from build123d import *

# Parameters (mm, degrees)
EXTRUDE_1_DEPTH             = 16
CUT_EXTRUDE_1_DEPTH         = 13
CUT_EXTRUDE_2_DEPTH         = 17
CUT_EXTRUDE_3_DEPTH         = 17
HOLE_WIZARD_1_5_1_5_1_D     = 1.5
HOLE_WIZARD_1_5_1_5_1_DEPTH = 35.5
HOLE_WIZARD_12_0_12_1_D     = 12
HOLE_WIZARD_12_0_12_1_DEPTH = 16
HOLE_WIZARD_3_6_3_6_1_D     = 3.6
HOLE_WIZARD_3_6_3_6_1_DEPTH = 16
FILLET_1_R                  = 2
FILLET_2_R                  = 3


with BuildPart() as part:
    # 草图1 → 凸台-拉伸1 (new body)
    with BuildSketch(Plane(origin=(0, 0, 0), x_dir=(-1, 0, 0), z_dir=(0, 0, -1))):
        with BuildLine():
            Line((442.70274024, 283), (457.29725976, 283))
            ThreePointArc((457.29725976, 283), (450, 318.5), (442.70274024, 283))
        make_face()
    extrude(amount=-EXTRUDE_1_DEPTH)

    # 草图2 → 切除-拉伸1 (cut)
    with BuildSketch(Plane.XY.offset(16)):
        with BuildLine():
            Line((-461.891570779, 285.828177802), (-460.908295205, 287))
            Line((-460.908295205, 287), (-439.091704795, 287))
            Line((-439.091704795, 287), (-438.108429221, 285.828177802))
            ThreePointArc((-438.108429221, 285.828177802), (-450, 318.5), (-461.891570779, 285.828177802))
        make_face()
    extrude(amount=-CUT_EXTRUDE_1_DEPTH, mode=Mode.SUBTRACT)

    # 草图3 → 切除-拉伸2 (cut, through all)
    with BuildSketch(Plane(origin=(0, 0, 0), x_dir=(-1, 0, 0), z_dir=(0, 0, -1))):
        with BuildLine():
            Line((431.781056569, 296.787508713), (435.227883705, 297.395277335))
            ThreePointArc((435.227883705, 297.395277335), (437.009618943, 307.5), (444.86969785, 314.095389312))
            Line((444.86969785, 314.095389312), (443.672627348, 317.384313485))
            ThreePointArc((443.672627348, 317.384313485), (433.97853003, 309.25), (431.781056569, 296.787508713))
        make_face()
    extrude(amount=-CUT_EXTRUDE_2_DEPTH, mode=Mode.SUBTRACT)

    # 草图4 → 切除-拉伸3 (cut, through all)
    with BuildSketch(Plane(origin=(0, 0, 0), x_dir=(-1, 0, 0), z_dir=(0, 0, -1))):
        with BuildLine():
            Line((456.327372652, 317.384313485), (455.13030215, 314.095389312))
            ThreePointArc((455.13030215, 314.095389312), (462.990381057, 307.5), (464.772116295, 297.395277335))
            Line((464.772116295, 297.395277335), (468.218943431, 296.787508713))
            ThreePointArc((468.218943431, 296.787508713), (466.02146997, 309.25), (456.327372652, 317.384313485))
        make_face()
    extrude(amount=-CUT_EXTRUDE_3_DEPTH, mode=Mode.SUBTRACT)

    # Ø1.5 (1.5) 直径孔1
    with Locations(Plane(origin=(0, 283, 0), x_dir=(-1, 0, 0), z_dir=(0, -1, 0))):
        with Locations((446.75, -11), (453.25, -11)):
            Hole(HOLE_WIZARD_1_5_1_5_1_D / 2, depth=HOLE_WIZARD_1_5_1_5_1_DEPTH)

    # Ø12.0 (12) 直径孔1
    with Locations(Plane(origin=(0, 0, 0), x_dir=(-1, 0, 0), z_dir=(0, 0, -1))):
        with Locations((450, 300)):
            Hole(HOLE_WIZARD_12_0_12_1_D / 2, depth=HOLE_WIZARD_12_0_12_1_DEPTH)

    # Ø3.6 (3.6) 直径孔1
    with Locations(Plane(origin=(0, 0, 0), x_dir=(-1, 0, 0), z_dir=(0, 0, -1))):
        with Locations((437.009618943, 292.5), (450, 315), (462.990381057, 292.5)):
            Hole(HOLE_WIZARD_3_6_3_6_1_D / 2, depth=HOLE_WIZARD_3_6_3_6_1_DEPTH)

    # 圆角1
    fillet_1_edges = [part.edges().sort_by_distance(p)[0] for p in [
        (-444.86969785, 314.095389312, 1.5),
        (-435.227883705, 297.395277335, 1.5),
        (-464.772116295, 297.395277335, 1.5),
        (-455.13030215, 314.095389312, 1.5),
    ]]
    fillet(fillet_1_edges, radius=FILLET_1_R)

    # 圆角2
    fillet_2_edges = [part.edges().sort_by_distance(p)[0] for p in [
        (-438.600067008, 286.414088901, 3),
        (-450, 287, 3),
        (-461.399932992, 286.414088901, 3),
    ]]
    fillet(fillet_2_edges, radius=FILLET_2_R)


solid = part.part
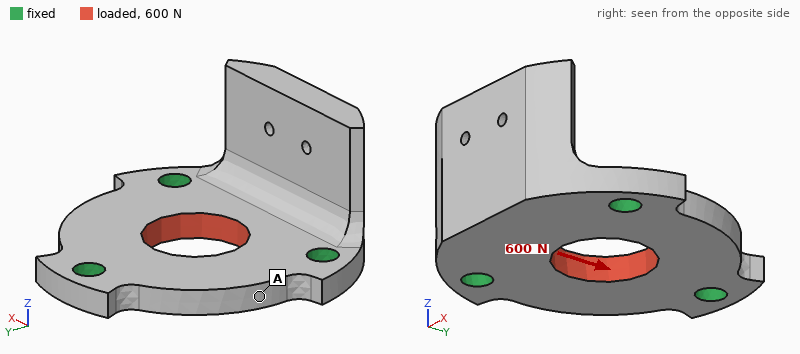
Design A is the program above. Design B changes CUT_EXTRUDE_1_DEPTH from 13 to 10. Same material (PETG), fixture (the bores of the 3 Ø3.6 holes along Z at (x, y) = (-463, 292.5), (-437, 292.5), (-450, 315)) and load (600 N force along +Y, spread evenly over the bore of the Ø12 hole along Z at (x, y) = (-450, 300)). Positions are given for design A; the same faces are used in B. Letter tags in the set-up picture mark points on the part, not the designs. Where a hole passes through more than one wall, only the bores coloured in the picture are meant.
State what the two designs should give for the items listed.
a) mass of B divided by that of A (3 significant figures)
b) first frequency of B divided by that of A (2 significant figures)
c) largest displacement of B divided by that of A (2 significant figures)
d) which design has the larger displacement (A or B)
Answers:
1.60
2.3
0.52
A
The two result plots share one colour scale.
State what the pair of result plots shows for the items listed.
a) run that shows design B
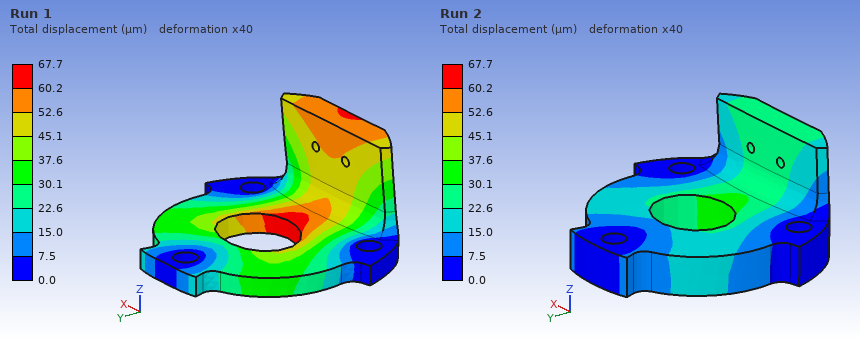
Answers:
Run 2
